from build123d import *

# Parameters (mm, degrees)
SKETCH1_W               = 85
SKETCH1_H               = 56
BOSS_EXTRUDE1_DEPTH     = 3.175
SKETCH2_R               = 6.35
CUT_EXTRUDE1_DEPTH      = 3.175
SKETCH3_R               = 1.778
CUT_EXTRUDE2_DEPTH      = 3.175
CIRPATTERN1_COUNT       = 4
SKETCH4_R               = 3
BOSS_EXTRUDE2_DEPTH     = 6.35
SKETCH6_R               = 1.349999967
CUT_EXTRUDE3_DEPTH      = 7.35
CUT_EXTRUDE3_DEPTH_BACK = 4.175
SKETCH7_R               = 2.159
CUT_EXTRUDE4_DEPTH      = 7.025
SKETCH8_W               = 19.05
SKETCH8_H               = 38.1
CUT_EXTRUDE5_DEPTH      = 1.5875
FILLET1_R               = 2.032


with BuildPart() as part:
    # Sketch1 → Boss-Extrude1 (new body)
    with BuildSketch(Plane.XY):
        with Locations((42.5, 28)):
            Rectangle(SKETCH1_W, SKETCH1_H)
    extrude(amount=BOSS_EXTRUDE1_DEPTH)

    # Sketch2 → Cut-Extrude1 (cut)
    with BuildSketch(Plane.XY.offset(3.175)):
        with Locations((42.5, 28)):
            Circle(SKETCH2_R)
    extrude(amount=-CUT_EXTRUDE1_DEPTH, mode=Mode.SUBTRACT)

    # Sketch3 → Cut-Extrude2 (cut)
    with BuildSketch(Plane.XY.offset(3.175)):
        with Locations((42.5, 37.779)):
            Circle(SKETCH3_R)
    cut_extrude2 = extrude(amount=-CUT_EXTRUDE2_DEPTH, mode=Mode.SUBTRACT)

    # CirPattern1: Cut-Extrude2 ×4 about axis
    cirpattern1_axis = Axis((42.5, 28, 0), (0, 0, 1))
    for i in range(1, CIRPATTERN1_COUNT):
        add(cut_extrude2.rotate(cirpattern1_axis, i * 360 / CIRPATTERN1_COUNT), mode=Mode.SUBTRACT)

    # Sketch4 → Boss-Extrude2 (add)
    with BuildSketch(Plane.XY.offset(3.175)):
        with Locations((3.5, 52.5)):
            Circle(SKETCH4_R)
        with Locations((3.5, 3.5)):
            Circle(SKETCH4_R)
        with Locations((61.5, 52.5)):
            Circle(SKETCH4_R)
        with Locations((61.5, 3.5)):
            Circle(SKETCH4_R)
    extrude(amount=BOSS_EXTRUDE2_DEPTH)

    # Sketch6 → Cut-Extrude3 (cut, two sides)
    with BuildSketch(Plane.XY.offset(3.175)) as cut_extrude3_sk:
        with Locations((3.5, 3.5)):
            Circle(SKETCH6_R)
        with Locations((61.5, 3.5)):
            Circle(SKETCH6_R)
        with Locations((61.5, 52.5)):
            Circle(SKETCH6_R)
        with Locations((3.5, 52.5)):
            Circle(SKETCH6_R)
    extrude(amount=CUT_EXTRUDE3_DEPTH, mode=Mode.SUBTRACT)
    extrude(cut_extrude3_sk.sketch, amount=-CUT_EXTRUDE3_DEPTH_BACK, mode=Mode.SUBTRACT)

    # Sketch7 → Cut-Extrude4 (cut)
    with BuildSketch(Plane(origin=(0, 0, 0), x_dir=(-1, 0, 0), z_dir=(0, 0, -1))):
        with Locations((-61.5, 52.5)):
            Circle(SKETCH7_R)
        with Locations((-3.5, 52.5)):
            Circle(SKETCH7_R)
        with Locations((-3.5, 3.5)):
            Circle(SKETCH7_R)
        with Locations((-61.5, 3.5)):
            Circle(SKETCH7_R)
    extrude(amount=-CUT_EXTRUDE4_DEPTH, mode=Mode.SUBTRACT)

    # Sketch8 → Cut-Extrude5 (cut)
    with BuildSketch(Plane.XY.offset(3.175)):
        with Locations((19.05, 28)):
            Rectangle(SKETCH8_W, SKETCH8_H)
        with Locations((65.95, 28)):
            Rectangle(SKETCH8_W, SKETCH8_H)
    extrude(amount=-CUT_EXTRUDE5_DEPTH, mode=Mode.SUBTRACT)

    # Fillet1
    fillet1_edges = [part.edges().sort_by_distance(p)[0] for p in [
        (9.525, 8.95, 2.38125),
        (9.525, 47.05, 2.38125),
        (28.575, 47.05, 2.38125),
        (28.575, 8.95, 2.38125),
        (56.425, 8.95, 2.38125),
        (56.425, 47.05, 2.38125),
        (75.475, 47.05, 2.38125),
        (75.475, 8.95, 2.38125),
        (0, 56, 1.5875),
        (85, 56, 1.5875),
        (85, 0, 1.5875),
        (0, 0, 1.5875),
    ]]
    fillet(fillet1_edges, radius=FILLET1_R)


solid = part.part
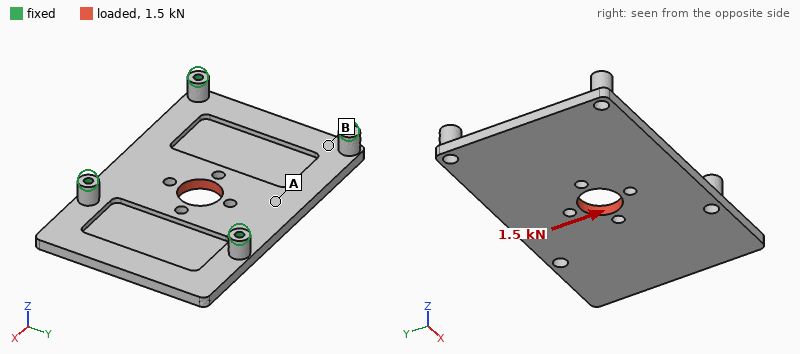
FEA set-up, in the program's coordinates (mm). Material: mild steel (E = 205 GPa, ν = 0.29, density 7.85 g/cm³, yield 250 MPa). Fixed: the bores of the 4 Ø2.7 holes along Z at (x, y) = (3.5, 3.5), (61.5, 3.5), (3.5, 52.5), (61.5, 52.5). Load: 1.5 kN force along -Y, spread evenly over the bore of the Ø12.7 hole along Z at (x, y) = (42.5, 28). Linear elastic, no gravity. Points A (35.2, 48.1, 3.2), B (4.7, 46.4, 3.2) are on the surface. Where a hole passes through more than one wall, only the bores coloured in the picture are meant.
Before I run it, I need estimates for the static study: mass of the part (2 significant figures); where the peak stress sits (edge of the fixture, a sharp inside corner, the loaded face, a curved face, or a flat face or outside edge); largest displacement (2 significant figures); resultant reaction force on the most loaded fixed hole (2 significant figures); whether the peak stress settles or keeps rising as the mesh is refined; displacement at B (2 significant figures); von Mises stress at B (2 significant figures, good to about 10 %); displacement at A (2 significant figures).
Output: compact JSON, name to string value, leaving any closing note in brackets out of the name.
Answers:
{"mass of the part": "98 g", "where the peak stress sits": "edge of the fixture", "largest displacement": "12 µm", "resultant reaction force on the most loaded fixed hole": "460 N", "whether the peak stress settles or keeps rising as the mesh is refined": "keeps rising", "displacement at B": "6.2 µm", "von Mises stress at B": "25 MPa", "displacement at A": "11 µm"}
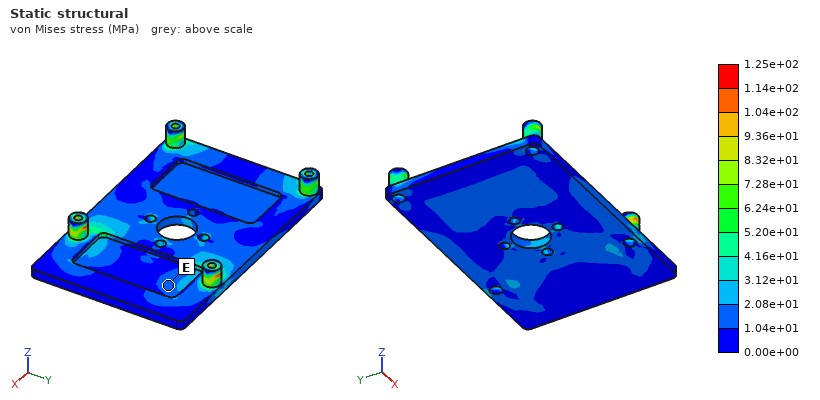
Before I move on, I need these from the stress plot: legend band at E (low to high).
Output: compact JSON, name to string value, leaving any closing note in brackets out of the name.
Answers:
{"legend band at E": "1.04e+01 to 2.08e+01 MPa"}
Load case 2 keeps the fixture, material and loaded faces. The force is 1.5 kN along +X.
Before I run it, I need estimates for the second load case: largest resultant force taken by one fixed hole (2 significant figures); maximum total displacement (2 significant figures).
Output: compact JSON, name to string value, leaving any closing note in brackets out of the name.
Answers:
{"largest resultant force taken by one fixed hole": "400 N", "maximum total displacement": "25 µm"}
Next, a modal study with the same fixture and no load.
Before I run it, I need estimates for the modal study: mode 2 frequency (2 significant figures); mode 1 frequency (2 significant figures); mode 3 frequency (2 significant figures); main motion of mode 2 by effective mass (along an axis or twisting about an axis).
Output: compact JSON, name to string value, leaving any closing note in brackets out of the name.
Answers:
{"mode 2 frequency": "3100 Hz", "mode 1 frequency": "2400 Hz", "mode 3 frequency": "4500 Hz", "main motion of mode 2 by effective mass": "along Z"}
